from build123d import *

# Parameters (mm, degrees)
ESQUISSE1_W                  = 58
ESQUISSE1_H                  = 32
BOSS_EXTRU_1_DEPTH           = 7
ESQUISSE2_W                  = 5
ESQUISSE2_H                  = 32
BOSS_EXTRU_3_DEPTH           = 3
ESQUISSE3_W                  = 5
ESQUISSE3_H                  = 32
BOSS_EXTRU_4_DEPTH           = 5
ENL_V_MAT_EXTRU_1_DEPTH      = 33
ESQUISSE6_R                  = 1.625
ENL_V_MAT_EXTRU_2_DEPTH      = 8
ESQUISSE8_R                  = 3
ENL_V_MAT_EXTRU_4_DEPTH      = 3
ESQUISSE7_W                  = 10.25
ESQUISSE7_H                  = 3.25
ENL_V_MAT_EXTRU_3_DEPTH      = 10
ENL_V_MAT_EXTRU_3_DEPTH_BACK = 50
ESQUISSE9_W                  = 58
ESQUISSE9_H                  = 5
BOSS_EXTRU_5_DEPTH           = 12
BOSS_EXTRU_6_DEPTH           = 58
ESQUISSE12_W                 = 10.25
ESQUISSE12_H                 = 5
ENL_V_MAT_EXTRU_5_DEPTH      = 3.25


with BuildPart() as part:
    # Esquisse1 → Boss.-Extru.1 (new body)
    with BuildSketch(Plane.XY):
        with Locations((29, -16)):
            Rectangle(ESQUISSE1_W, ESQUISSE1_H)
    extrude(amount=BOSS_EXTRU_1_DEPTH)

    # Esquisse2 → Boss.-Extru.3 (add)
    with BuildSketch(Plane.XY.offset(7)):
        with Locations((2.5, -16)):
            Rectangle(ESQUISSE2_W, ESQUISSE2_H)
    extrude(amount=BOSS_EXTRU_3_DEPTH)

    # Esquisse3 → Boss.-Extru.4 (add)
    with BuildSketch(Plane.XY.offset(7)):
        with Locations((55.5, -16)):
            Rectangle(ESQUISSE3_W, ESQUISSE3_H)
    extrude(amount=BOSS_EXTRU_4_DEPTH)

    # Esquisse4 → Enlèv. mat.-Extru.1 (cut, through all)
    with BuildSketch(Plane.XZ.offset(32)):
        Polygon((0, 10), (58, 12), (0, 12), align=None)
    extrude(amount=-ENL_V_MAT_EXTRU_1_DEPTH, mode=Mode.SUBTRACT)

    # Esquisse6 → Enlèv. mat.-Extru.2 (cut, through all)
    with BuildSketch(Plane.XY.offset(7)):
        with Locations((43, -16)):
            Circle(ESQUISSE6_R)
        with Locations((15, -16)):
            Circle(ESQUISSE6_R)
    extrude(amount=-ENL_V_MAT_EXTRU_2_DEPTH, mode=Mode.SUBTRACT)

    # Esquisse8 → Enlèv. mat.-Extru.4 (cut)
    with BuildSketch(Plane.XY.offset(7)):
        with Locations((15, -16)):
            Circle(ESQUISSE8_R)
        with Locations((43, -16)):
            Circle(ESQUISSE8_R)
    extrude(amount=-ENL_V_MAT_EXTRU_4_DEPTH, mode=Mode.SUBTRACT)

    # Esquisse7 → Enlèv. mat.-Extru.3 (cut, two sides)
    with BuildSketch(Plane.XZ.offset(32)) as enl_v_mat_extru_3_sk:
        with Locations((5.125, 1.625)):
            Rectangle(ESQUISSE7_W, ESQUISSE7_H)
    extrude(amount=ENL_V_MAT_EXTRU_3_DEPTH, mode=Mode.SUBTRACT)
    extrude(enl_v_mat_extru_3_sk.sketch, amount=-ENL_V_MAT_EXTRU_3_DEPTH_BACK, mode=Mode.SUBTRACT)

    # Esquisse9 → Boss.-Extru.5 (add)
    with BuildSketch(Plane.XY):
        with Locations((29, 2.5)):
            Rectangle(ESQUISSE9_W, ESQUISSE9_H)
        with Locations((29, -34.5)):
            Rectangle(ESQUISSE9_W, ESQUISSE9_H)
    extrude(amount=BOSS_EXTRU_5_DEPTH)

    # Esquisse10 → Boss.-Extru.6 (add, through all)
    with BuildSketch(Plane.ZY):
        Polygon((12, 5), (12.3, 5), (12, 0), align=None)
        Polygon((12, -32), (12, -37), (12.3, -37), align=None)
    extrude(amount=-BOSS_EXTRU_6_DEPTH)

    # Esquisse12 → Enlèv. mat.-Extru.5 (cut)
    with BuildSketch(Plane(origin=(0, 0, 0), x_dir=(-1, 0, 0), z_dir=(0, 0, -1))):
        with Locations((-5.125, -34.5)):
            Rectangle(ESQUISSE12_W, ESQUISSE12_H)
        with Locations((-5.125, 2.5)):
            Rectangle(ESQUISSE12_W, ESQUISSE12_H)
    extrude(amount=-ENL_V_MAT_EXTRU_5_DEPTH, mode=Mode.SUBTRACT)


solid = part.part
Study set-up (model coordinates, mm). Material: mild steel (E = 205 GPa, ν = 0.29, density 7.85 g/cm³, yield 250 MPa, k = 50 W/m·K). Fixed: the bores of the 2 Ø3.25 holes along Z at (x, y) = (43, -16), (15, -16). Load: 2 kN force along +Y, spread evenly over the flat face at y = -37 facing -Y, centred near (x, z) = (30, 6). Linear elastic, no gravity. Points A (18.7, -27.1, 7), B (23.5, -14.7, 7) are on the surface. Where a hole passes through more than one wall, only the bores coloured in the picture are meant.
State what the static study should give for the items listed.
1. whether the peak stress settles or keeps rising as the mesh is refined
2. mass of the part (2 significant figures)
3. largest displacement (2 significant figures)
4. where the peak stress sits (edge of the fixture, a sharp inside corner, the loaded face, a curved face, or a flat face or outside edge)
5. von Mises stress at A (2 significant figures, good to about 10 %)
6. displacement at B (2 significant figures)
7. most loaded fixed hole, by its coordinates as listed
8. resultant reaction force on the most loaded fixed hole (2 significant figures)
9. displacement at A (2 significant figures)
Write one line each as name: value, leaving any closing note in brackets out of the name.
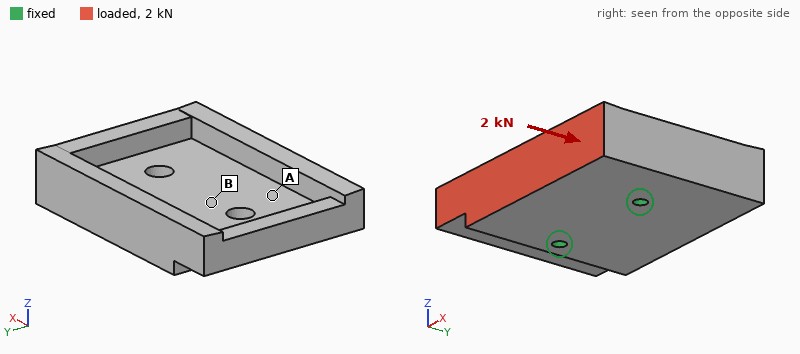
whether the peak stress settles or keeps rising as the mesh is refined: keeps rising
mass of the part: 150 g
largest displacement: 15 µm
where the peak stress sits: edge of the fixture
von Mises stress at A: 15 MPa
displacement at B: 2.8 µm
most loaded fixed hole, by its coordinates as listed: (43, -16)
resultant reaction force on the most loaded fixed hole: 1.1 kN
displacement at A: 6.9 µm
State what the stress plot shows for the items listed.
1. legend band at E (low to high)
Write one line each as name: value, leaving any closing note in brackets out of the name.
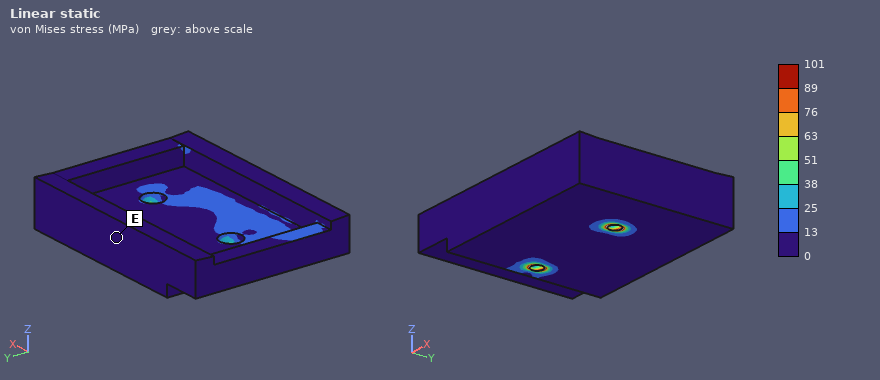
legend band at E: 0 to 13 MPa
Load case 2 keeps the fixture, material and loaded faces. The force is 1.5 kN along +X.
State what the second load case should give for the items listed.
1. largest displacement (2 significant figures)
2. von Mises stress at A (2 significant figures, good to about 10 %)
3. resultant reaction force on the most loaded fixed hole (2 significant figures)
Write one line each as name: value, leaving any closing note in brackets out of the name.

largest displacement: 5.1 µm
von Mises stress at A: 15 MPa
resultant reaction force on the most loaded fixed hole: 1.4 kN
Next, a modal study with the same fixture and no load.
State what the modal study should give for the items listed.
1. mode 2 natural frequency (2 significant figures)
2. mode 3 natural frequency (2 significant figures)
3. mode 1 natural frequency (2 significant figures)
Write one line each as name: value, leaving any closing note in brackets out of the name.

mode 2 natural frequency: 8100 Hz
mode 3 natural frequency: 9000 Hz
mode 1 natural frequency: 3800 Hz
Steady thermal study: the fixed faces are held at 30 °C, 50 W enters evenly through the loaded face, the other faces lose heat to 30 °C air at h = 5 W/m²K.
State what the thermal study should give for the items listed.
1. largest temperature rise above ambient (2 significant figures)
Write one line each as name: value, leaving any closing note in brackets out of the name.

largest temperature rise above ambient: 75 K
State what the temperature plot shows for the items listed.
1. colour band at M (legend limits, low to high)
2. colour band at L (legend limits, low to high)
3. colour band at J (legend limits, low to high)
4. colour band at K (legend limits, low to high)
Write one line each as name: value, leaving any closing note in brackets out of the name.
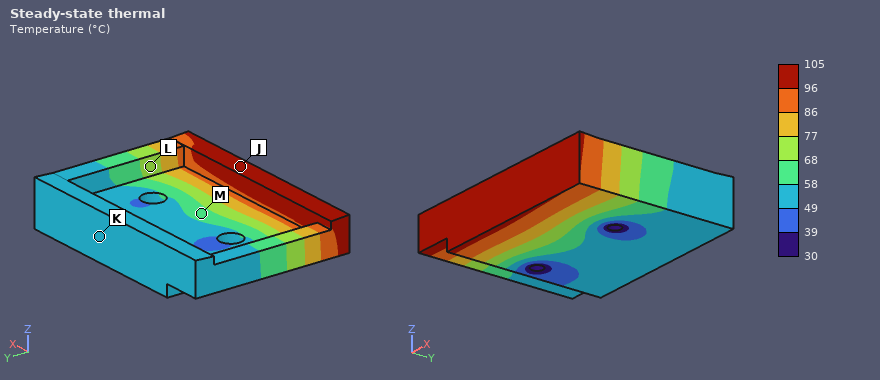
colour band at M: 58 to 68 °C
colour band at L: 68 to 77 °C
colour band at J: 96 to 105 °C
colour band at K: 49 to 58 °C
